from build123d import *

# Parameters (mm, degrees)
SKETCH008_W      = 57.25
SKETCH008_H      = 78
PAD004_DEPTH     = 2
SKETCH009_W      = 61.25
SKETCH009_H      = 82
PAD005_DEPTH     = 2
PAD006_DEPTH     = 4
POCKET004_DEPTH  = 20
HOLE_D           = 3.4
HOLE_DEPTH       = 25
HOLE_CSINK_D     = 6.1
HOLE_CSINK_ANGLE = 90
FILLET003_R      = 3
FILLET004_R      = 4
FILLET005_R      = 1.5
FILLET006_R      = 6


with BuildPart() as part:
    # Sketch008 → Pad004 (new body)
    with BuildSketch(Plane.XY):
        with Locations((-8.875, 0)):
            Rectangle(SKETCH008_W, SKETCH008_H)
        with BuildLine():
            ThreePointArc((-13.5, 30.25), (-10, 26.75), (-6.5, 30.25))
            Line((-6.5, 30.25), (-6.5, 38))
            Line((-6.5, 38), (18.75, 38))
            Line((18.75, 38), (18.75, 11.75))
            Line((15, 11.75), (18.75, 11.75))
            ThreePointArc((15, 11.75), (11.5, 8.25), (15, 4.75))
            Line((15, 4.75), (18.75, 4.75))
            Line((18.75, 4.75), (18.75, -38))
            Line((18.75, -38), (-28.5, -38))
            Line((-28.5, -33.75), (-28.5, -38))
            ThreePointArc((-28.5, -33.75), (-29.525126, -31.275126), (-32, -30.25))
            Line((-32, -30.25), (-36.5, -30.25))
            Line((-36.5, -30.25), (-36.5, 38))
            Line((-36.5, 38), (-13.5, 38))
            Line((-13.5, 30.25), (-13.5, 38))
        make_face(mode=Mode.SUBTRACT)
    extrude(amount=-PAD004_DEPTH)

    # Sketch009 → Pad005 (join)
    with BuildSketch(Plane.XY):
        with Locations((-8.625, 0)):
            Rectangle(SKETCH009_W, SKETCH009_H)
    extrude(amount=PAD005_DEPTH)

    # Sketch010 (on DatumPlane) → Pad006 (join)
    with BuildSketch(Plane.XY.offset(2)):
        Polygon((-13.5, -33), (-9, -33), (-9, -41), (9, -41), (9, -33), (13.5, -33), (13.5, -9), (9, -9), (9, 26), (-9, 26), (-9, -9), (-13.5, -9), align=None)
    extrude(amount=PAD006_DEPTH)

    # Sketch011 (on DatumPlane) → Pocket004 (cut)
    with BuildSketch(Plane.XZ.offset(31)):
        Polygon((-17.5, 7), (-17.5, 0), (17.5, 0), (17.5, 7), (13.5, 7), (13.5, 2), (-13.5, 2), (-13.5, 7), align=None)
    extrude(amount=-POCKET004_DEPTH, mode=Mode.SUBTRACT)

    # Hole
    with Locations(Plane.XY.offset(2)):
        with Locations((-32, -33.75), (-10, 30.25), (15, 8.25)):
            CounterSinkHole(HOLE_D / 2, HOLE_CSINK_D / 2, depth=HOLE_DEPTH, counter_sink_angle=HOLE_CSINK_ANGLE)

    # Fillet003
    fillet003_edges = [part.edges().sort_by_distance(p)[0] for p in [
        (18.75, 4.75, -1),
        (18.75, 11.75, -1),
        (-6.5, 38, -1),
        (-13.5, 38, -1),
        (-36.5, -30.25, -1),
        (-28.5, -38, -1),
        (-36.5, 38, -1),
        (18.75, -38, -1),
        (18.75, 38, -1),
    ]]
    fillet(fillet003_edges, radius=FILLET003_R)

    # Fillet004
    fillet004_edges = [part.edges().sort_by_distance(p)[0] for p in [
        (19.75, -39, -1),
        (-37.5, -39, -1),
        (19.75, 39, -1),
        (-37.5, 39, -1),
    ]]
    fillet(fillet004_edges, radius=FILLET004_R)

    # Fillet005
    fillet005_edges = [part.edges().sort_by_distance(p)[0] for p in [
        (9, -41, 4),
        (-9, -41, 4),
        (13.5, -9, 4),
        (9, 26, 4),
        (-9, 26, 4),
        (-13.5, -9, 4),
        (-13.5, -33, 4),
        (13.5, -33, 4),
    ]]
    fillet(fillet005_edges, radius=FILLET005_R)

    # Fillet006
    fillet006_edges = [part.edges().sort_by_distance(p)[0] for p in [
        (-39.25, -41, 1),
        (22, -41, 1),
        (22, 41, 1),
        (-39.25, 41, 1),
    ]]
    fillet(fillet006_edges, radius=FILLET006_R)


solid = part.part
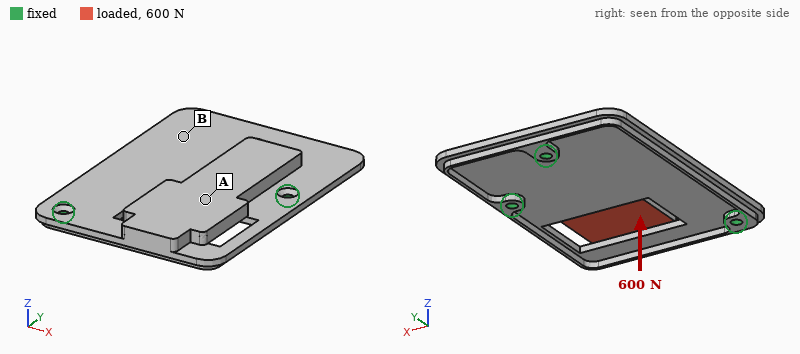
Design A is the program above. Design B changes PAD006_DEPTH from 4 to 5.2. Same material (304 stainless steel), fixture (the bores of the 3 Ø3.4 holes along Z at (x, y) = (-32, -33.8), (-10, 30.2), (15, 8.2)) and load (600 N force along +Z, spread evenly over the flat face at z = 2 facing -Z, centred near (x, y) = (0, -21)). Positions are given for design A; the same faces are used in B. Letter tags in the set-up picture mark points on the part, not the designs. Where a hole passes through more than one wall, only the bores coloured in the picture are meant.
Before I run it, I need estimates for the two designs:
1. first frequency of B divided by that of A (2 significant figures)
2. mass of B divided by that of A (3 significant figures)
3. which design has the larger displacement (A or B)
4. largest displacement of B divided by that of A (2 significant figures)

1.00
1.11
A
0.78
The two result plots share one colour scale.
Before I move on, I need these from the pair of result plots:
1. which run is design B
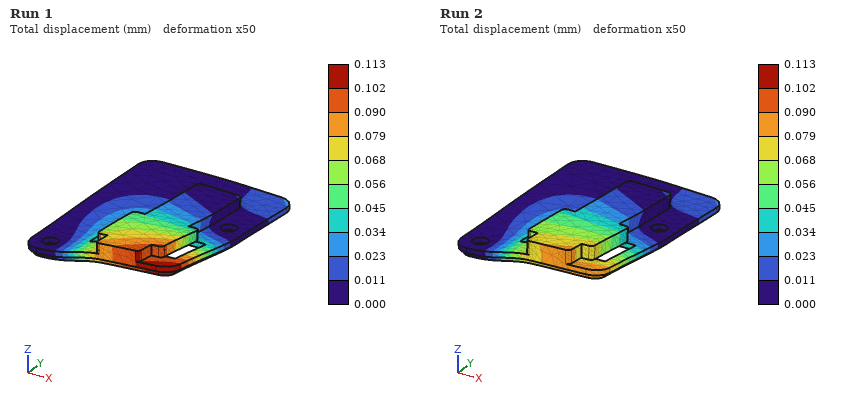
Run 2
